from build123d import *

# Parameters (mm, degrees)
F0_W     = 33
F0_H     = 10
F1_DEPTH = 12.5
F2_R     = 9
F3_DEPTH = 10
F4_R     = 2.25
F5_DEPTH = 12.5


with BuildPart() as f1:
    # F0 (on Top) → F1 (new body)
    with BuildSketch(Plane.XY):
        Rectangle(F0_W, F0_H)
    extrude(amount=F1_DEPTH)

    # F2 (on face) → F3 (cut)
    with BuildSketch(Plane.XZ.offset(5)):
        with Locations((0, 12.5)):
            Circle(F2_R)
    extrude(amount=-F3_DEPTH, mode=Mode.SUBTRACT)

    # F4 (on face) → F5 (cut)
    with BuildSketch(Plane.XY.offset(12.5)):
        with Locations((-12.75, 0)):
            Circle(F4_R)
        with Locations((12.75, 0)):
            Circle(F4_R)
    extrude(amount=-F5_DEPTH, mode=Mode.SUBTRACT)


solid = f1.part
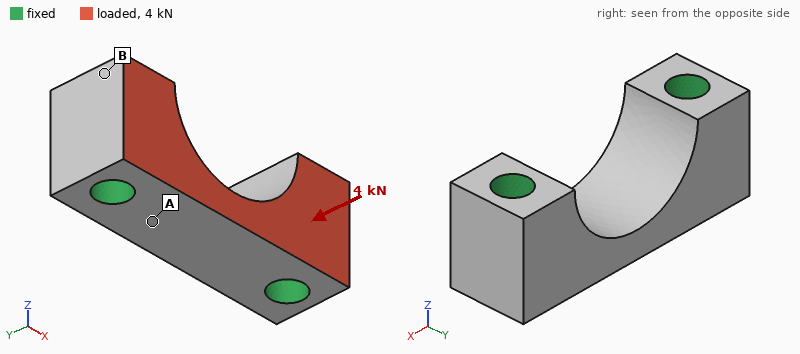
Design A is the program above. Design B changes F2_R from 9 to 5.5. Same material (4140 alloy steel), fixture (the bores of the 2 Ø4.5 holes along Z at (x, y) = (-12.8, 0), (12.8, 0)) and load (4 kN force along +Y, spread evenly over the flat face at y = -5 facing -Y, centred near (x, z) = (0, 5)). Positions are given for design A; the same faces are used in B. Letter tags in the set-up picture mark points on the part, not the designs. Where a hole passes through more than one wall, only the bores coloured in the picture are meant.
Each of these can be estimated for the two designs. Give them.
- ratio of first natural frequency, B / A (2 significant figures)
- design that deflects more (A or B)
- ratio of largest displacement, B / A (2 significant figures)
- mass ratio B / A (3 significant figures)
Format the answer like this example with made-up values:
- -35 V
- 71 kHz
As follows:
- 0.92
- A
- 0.88
- 1.32
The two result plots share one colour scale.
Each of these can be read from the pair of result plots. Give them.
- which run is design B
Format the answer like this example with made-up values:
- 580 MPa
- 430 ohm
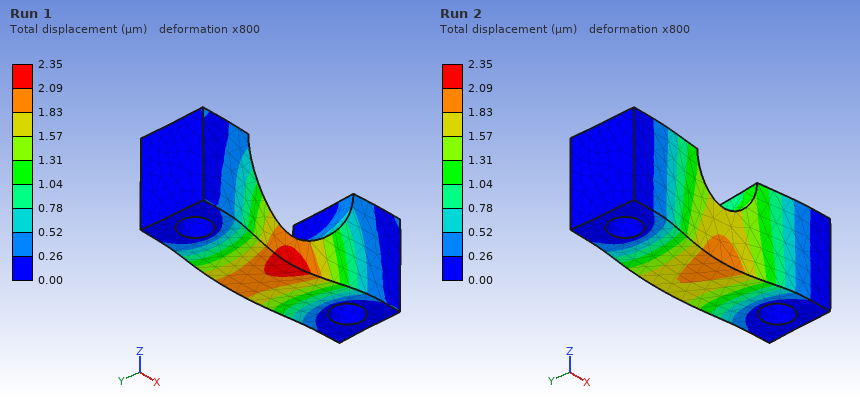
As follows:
- Run 2
